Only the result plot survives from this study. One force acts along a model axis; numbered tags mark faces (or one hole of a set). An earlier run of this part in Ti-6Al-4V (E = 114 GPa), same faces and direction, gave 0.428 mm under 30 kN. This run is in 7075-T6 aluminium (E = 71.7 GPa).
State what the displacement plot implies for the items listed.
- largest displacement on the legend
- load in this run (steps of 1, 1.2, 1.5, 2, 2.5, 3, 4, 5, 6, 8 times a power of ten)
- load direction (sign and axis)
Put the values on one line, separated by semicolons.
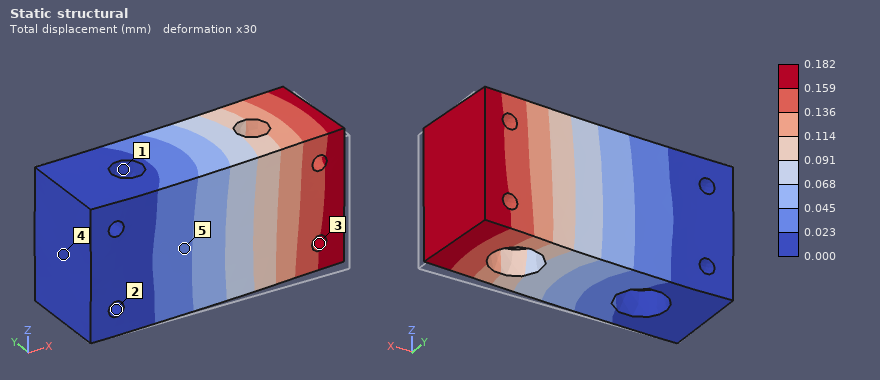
0.182 mm; 8 kN; +Y
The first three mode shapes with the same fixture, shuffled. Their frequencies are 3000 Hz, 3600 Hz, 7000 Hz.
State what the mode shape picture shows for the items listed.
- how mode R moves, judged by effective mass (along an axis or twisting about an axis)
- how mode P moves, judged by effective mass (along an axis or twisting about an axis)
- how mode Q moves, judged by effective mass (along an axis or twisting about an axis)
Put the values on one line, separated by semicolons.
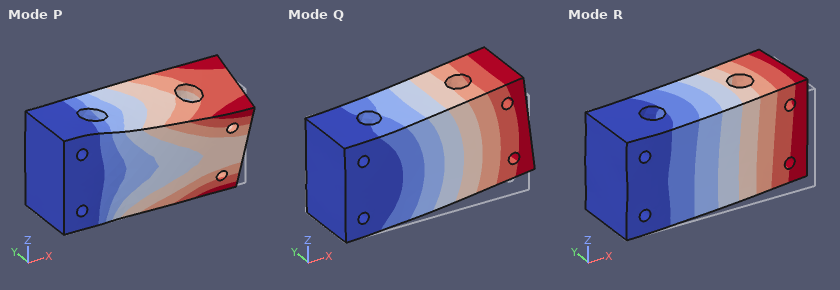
along Y; twisting about X; along Z
